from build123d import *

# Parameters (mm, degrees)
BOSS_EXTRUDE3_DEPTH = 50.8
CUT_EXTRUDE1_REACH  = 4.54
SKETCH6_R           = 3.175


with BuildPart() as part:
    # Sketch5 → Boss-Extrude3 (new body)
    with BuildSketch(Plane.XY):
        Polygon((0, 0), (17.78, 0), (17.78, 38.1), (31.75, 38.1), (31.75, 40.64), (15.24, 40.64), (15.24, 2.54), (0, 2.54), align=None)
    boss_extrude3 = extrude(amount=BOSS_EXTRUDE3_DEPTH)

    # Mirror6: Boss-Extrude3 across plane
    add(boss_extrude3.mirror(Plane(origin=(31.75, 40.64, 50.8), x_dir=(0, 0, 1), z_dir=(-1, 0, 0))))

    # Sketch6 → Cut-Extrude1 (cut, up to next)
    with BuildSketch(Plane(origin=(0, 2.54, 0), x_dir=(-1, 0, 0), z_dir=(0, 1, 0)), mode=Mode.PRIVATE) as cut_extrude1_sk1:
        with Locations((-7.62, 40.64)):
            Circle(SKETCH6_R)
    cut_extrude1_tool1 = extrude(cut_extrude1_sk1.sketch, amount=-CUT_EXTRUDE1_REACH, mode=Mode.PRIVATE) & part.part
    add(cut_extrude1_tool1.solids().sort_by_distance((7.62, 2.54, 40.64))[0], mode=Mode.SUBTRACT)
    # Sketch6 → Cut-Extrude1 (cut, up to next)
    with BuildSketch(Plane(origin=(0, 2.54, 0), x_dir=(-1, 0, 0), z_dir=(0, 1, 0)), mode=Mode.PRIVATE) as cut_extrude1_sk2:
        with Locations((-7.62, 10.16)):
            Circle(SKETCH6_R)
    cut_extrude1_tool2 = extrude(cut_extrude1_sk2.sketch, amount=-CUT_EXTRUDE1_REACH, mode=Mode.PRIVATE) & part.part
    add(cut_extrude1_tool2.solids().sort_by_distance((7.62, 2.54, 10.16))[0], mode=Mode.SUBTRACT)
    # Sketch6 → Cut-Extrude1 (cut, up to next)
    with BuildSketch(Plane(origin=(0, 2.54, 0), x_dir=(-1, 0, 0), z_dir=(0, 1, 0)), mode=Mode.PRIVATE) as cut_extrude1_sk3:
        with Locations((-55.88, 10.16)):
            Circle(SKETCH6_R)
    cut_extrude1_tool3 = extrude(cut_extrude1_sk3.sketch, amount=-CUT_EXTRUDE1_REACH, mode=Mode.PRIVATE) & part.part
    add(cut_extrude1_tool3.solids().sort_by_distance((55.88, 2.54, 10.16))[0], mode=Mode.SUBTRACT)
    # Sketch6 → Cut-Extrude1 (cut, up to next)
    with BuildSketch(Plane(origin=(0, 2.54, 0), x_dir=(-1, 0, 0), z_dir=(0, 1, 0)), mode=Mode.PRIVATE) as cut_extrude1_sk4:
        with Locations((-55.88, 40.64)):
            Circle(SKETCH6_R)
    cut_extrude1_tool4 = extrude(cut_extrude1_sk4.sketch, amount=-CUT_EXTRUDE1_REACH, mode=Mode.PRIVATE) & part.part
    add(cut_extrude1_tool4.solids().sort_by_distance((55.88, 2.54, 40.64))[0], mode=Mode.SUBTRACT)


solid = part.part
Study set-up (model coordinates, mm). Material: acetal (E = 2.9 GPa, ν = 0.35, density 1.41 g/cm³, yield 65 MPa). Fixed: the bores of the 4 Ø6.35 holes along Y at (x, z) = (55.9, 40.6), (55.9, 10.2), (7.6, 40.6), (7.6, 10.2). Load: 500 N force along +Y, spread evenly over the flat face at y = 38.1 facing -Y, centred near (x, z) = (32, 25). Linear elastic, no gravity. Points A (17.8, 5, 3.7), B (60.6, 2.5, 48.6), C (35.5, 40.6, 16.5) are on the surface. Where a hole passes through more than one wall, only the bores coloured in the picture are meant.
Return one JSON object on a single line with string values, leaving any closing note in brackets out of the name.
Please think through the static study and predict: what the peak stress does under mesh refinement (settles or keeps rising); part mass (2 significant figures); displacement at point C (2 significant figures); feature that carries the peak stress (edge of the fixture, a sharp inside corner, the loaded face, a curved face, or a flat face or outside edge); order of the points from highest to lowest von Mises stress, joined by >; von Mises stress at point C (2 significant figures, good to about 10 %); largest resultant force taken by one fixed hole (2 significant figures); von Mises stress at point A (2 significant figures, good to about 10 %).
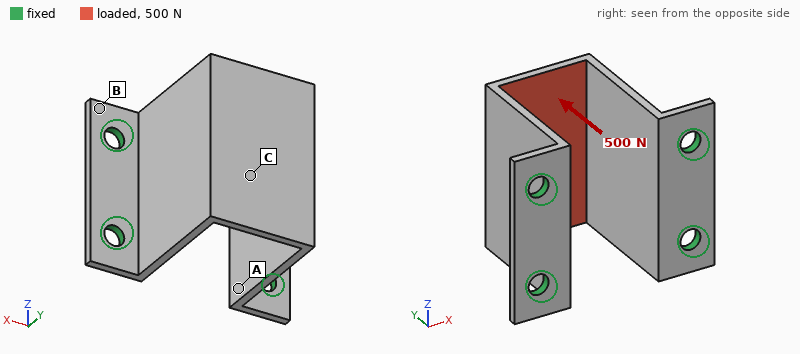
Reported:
{"what the peak stress does under mesh refinement": "keeps rising", "part mass": "25 g", "displacement at point C": "0.50 mm", "feature that carries the peak stress": "edge of the fixture", "order of the points from highest to lowest von Mises stress, joined by >": "C > A > B", "von Mises stress at point C": "16 MPa", "largest resultant force taken by one fixed hole": "130 N", "von Mises stress at point A": "7.3 MPa"}
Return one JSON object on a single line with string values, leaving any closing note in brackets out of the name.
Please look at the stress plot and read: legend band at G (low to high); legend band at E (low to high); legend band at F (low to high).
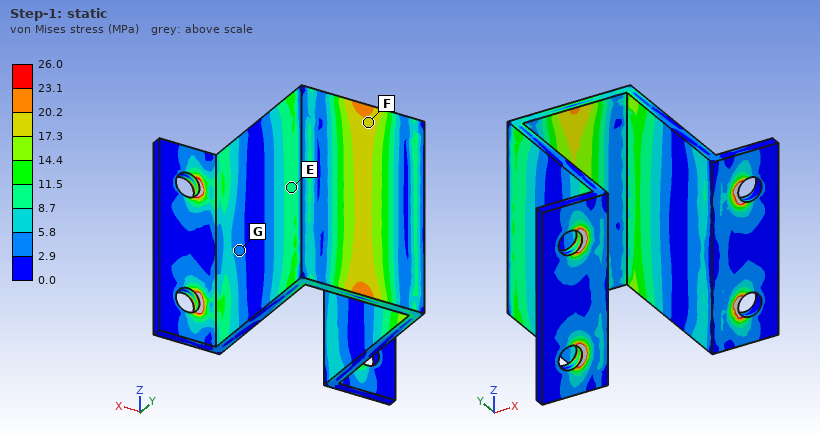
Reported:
{"legend band at G": "2.9 to 5.8 MPa", "legend band at E": "8.7 to 11.5 MPa", "legend band at F": "17.3 to 20.2 MPa"}
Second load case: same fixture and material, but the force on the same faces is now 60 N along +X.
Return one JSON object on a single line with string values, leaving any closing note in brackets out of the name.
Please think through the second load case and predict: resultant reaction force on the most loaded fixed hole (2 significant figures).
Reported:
{"resultant reaction force on the most loaded fixed hole": "24 N"}
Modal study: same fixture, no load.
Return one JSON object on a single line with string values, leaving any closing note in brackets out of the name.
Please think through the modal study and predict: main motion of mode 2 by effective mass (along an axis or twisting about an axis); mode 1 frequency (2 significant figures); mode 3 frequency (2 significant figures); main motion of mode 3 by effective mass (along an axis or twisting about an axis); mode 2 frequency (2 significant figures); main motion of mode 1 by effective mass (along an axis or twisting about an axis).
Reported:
{"main motion of mode 2 by effective mass": "twisting about Y", "mode 1 frequency": "370 Hz", "mode 3 frequency": "1000 Hz", "main motion of mode 3 by effective mass": "along Z", "mode 2 frequency": "840 Hz", "main motion of mode 1 by effective mass": "along X"}
